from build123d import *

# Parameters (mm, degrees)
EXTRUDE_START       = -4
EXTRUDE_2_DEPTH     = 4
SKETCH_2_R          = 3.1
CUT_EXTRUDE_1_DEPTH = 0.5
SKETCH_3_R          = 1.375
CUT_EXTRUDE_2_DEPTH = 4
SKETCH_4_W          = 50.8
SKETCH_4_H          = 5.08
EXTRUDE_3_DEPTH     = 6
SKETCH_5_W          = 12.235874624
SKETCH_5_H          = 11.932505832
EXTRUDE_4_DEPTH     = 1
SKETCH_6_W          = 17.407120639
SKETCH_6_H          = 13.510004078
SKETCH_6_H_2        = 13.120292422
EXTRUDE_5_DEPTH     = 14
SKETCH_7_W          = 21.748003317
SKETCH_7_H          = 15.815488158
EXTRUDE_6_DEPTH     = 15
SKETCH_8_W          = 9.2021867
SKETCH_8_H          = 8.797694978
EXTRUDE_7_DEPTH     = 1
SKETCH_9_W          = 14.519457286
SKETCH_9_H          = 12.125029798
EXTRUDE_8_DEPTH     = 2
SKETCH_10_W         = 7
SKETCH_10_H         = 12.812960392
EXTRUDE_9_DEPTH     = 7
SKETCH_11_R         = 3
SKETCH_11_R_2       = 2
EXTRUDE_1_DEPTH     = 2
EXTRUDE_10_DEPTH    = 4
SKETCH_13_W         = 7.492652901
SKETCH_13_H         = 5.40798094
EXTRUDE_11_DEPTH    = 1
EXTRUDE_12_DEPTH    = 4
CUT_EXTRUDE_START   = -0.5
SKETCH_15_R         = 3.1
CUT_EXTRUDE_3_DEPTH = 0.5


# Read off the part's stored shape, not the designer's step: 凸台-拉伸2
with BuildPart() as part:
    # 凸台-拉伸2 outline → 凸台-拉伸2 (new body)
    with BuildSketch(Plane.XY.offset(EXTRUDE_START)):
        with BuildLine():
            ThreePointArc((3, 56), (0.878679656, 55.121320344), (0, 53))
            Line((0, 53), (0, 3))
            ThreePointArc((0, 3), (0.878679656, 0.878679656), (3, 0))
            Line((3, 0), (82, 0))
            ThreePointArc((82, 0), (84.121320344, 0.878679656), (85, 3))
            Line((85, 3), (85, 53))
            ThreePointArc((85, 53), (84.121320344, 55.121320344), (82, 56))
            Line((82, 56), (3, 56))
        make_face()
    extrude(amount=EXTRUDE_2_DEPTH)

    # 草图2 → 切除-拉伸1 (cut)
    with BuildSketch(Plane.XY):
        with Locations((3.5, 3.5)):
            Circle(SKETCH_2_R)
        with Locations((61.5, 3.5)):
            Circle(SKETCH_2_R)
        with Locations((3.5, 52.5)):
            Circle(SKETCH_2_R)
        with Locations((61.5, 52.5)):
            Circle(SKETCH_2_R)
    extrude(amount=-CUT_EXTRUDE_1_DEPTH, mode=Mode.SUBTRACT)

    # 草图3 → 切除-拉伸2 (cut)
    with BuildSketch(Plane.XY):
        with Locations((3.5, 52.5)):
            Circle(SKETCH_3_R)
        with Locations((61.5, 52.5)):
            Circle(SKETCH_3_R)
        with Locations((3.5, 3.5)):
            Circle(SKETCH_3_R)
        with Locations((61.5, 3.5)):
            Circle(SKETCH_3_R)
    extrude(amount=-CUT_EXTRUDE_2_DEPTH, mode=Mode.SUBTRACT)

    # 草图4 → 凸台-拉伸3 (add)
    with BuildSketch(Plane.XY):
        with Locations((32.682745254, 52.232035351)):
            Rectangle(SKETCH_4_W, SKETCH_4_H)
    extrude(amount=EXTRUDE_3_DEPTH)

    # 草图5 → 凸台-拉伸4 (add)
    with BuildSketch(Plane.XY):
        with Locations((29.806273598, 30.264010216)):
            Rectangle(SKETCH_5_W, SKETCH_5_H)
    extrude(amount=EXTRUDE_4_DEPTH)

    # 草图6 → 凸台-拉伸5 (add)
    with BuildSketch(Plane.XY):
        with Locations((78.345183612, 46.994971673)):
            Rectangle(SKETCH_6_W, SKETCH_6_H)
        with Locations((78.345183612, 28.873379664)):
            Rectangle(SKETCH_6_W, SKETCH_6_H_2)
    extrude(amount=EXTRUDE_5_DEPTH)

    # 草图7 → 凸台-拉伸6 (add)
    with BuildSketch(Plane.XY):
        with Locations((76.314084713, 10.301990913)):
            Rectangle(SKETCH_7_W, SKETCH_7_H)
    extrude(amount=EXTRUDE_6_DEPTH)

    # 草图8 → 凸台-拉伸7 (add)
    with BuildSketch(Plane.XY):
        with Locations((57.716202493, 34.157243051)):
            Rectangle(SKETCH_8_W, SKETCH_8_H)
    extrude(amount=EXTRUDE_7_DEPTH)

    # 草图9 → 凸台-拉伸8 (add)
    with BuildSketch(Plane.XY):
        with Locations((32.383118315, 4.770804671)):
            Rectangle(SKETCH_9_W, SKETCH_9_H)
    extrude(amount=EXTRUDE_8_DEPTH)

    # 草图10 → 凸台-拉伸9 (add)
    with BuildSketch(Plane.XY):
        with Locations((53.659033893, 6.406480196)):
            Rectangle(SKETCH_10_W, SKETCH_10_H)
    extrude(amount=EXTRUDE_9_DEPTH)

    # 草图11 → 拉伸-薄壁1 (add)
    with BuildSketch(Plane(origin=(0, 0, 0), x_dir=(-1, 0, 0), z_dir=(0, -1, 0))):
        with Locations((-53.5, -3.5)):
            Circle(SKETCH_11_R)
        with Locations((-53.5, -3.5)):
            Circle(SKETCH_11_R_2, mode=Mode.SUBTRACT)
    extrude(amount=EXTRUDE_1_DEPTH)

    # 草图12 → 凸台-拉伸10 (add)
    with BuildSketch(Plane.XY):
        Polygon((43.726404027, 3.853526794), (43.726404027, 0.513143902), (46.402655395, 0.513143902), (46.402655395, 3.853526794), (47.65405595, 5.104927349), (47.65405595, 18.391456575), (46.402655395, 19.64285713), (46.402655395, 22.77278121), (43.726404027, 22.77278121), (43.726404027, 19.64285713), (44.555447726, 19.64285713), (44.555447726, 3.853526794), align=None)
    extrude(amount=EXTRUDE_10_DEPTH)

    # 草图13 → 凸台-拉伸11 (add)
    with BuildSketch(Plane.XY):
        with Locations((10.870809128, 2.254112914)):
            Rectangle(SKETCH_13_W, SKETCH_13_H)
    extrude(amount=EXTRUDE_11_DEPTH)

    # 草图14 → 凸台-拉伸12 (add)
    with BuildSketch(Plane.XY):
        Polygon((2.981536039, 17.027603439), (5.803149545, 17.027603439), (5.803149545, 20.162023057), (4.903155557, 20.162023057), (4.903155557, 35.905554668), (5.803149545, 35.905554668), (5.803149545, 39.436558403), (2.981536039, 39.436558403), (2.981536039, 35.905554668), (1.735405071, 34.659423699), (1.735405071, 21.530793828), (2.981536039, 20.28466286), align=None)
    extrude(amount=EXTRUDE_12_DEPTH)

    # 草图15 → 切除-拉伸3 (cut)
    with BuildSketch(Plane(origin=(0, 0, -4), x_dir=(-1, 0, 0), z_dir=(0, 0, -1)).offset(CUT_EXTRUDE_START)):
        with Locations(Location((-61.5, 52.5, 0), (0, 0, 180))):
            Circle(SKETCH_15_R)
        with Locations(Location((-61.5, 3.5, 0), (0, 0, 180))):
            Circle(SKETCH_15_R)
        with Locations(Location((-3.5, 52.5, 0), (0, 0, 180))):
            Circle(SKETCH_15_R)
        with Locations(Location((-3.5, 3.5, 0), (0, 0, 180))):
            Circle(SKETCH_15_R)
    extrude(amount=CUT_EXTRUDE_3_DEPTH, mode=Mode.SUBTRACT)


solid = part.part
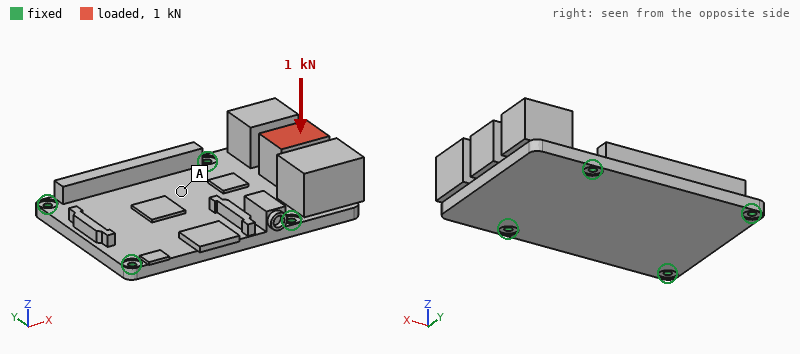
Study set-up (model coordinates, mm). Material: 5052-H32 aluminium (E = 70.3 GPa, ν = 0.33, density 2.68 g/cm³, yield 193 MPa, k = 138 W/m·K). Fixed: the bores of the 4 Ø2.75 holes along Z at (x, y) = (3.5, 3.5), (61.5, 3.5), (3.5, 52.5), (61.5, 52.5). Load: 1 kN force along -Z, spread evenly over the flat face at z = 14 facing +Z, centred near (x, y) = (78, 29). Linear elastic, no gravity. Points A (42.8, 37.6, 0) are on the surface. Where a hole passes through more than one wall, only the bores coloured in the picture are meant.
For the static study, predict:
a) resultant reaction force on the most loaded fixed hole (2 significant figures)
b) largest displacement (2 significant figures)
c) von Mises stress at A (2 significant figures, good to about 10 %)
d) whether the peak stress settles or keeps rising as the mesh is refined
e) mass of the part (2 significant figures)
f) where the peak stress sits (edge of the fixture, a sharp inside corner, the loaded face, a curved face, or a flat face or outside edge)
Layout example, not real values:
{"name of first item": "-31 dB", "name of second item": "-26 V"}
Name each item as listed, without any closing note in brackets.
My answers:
{"resultant reaction force on the most loaded fixed hole": "630 N", "largest displacement": "0.36 mm", "von Mises stress at A": "23 MPa", "whether the peak stress settles or keeps rising as the mesh is refined": "keeps rising", "mass of the part": "91 g", "where the peak stress sits": "edge of the fixture"}
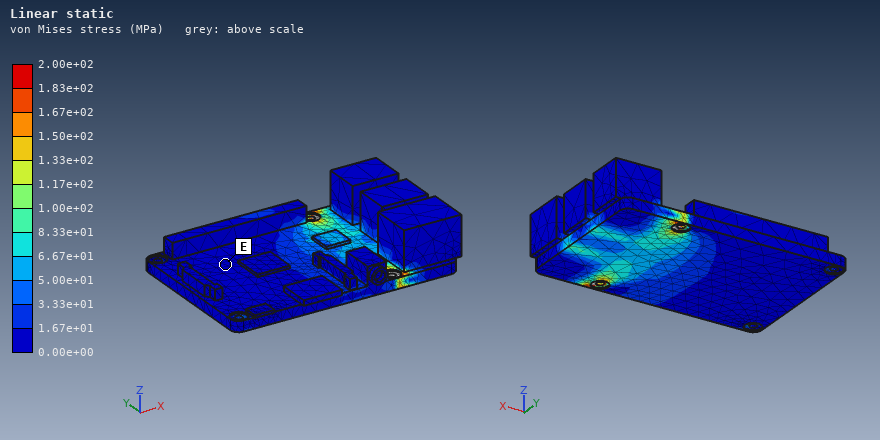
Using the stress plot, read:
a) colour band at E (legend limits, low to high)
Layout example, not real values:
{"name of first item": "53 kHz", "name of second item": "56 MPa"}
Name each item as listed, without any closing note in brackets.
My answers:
{"colour band at E": "0.00e+00 to 1.67e+01 MPa"}
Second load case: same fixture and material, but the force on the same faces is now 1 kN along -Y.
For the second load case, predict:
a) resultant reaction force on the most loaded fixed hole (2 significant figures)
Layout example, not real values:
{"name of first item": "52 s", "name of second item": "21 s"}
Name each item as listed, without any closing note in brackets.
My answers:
{"resultant reaction force on the most loaded fixed hole": "700 N"}
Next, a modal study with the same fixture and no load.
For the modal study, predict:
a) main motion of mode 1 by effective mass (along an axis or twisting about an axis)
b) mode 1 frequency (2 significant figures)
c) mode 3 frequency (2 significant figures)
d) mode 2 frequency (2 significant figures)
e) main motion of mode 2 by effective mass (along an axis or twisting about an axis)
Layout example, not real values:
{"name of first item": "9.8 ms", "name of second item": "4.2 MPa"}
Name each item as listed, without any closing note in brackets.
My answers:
{"main motion of mode 1 by effective mass": "along Z", "mode 1 frequency": "1700 Hz", "mode 3 frequency": "4500 Hz", "mode 2 frequency": "4200 Hz", "main motion of mode 2 by effective mass": "along Z"}
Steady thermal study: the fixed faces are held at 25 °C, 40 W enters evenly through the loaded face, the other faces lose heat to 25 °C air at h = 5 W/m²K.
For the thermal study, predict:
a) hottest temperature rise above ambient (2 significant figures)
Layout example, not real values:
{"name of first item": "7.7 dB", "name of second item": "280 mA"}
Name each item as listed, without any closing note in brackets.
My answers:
{"hottest temperature rise above ambient": "56 K"}
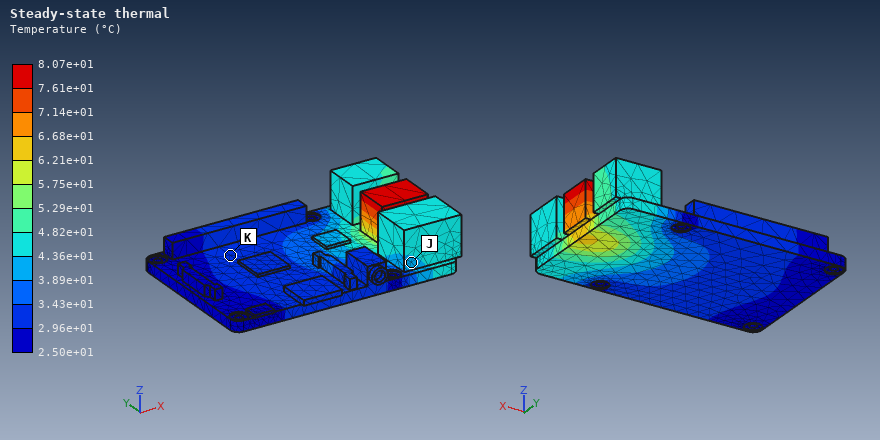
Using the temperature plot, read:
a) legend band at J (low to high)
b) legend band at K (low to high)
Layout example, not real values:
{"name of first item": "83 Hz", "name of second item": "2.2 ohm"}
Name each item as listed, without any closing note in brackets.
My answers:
{"legend band at J": "3.89e+01 to 4.36e+01 °C", "legend band at K": "2.96e+01 to 3.43e+01 °C"}
